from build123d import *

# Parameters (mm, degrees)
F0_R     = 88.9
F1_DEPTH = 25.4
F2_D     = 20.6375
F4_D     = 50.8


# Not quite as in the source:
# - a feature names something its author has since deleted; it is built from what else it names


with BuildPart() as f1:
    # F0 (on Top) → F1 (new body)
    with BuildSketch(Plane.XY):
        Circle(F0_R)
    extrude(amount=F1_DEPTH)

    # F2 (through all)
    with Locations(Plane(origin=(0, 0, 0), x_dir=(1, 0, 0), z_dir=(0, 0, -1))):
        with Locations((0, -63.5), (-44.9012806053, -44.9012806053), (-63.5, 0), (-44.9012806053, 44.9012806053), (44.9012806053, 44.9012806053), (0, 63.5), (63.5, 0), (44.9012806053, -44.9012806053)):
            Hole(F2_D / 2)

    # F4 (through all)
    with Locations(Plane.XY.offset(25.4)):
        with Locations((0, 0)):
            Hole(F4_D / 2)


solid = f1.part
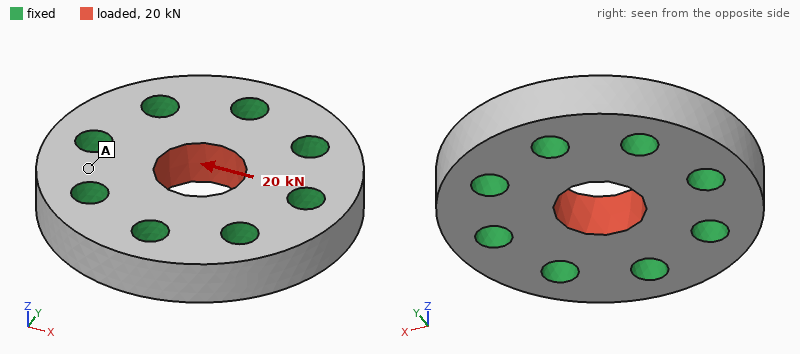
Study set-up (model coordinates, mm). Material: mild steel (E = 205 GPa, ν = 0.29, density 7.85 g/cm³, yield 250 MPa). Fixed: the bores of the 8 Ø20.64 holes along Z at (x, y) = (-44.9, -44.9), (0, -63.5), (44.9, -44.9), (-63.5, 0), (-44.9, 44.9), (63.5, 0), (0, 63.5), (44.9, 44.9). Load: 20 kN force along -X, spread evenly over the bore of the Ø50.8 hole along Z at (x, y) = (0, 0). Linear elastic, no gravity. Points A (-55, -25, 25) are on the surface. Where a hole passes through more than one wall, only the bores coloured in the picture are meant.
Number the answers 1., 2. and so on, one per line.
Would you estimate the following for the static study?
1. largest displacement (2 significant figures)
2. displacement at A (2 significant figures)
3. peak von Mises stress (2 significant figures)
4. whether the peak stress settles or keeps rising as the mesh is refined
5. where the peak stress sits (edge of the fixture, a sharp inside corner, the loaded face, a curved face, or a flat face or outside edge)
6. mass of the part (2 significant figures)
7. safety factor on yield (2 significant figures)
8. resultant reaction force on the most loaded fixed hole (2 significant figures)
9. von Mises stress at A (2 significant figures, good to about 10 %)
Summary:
1. 0.82 µm
2. 0.17 µm
3. 8.6 MPa
4. settles
5. the loaded face
6. 4.0 kg
7. 29
8. 4.1 kN
9. 1.5 MPa
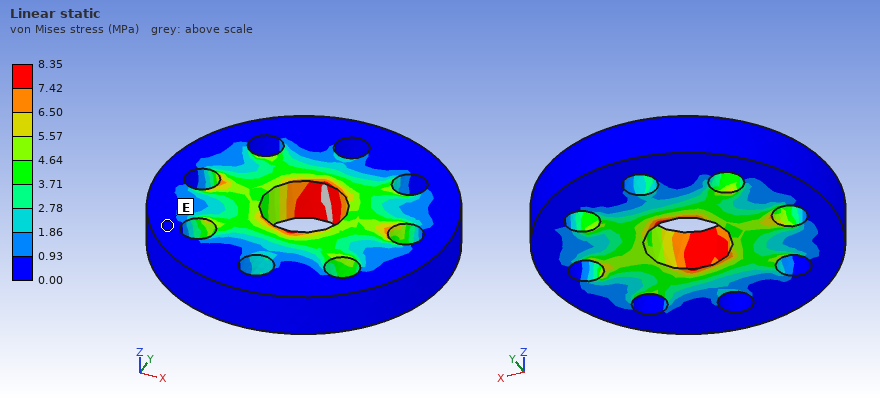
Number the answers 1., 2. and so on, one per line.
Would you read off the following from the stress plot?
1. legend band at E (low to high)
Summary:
1. 0.00 to 0.93 MPa
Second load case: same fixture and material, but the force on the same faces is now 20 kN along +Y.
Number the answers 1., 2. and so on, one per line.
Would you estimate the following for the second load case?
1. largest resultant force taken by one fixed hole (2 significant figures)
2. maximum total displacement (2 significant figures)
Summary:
1. 4.1 kN
2. 0.82 µm
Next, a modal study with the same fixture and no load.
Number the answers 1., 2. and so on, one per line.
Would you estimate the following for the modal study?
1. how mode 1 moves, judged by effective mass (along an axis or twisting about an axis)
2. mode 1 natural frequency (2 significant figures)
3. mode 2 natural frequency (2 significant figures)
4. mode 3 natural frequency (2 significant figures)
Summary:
1. along Z
2. 18 kHz
3. 22 kHz
4. 22 kHz
